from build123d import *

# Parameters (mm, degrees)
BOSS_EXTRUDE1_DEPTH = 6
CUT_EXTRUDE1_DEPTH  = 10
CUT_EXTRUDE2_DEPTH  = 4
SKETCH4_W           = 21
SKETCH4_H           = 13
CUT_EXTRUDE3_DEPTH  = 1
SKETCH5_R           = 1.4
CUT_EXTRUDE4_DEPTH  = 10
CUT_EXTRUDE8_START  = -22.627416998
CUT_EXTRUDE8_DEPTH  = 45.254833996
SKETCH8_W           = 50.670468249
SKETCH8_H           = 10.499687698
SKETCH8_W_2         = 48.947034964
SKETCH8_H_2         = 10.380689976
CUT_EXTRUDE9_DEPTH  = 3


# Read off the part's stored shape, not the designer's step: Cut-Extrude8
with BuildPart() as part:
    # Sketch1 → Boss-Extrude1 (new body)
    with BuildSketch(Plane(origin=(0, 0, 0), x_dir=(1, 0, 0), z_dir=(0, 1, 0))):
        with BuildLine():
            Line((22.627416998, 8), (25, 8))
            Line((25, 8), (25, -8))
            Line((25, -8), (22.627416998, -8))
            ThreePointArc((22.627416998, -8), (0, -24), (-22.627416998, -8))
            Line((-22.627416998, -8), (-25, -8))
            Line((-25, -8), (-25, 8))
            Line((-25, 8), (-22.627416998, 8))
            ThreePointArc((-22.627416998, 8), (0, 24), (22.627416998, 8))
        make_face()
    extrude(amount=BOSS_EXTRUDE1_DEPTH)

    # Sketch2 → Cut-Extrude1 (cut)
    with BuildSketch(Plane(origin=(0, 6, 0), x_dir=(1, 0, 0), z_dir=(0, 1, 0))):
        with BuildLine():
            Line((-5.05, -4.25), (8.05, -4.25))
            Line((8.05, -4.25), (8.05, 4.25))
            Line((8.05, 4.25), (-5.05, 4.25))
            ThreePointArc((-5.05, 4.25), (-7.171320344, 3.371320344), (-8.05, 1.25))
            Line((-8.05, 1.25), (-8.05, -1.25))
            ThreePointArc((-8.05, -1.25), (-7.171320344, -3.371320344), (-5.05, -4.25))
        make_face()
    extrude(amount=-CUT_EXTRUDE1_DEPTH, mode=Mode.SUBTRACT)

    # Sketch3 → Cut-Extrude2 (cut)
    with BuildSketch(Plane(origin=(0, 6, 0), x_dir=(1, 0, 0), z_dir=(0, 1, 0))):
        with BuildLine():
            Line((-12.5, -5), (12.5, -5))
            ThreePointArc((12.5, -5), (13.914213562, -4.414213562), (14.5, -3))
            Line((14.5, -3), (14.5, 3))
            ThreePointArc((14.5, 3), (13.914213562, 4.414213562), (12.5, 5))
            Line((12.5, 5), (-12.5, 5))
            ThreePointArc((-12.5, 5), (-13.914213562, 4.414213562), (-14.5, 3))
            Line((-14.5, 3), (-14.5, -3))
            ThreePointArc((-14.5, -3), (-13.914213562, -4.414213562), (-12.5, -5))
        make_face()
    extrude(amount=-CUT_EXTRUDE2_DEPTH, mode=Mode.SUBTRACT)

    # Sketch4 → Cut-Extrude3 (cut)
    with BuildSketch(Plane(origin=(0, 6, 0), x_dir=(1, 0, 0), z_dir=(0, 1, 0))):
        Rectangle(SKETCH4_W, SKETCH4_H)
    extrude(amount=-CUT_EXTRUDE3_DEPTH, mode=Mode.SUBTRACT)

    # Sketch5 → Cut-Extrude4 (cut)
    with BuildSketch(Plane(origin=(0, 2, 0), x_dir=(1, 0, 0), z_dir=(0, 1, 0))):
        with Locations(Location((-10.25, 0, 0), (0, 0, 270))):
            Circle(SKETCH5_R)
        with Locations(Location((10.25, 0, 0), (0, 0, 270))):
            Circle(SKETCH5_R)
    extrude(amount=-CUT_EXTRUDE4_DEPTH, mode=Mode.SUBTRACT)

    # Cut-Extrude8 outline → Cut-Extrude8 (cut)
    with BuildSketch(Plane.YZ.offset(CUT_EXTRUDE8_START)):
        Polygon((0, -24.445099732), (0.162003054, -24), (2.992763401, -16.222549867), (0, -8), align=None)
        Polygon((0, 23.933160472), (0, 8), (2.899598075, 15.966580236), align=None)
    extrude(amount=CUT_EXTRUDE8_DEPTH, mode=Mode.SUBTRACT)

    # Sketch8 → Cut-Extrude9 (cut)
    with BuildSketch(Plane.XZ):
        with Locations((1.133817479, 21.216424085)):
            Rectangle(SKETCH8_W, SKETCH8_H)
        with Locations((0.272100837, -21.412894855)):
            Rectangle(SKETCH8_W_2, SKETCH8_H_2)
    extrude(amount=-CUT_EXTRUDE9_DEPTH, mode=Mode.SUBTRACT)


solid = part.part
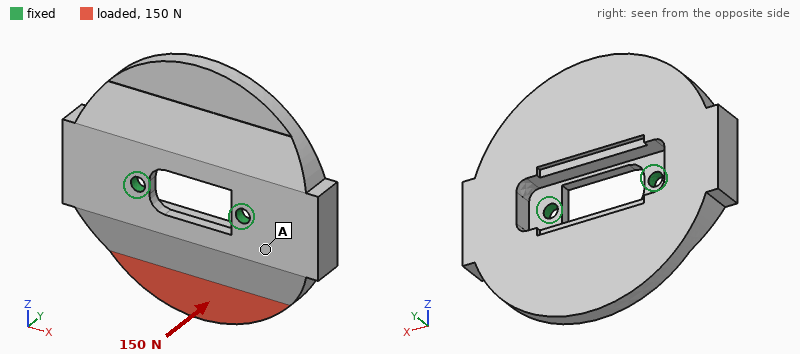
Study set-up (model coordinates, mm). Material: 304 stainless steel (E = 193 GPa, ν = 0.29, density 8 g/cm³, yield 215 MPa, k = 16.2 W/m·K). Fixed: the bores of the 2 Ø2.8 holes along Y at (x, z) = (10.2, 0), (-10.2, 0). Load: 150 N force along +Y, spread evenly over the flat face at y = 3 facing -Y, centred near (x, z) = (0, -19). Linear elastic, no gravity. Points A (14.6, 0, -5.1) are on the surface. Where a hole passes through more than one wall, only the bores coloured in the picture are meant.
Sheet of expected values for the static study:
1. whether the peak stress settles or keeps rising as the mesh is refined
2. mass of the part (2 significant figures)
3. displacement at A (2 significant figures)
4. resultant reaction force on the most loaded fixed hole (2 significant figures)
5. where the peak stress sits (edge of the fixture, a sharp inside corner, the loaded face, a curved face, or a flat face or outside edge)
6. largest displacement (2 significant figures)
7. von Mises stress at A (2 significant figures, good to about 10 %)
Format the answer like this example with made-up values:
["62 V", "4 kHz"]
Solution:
["keeps rising", "60 g", "6.6 µm", "76 N", "edge of the fixture", "42 µm", "28 MPa"]
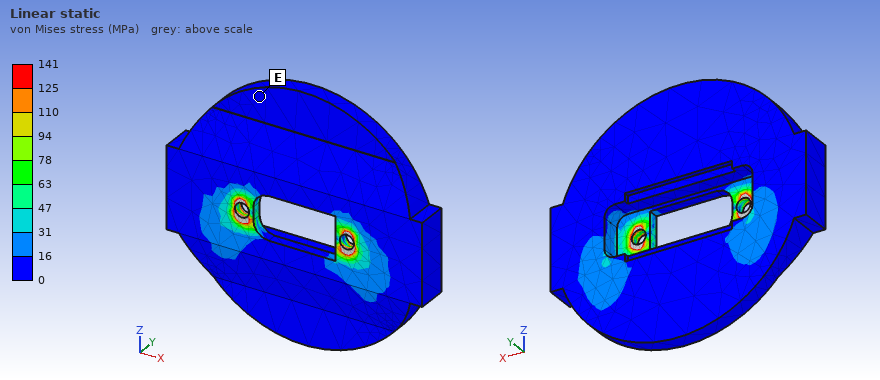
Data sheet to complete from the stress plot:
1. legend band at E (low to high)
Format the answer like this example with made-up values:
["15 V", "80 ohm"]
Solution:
["0 to 16 MPa"]
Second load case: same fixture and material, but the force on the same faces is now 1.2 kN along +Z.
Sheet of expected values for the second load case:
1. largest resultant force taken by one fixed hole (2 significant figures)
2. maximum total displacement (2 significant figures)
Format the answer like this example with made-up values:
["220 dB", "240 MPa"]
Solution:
["620 N", "28 µm"]
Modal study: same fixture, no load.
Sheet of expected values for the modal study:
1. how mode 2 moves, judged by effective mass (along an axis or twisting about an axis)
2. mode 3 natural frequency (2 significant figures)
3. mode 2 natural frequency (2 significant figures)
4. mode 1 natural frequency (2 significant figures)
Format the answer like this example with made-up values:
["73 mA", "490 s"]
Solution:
["along Y", "8000 Hz", "7400 Hz", "2600 Hz"]
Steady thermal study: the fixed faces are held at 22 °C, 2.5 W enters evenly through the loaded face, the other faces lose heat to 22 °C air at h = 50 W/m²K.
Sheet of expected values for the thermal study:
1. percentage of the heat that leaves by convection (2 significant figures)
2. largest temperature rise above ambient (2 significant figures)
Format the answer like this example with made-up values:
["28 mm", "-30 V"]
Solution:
["57 %", "25 K"]
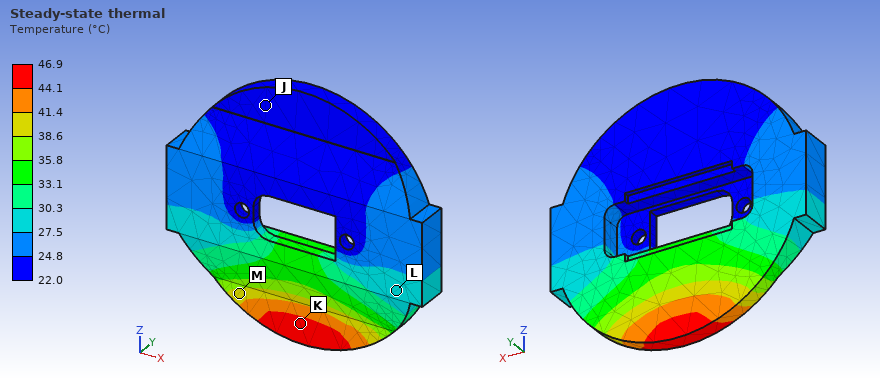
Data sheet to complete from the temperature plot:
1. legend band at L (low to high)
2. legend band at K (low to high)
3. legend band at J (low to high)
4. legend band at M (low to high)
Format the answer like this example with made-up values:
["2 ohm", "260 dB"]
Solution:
["27.5 to 30.3 °C", "44.1 to 46.9 °C", "22.0 to 24.8 °C", "38.6 to 41.4 °C"]
